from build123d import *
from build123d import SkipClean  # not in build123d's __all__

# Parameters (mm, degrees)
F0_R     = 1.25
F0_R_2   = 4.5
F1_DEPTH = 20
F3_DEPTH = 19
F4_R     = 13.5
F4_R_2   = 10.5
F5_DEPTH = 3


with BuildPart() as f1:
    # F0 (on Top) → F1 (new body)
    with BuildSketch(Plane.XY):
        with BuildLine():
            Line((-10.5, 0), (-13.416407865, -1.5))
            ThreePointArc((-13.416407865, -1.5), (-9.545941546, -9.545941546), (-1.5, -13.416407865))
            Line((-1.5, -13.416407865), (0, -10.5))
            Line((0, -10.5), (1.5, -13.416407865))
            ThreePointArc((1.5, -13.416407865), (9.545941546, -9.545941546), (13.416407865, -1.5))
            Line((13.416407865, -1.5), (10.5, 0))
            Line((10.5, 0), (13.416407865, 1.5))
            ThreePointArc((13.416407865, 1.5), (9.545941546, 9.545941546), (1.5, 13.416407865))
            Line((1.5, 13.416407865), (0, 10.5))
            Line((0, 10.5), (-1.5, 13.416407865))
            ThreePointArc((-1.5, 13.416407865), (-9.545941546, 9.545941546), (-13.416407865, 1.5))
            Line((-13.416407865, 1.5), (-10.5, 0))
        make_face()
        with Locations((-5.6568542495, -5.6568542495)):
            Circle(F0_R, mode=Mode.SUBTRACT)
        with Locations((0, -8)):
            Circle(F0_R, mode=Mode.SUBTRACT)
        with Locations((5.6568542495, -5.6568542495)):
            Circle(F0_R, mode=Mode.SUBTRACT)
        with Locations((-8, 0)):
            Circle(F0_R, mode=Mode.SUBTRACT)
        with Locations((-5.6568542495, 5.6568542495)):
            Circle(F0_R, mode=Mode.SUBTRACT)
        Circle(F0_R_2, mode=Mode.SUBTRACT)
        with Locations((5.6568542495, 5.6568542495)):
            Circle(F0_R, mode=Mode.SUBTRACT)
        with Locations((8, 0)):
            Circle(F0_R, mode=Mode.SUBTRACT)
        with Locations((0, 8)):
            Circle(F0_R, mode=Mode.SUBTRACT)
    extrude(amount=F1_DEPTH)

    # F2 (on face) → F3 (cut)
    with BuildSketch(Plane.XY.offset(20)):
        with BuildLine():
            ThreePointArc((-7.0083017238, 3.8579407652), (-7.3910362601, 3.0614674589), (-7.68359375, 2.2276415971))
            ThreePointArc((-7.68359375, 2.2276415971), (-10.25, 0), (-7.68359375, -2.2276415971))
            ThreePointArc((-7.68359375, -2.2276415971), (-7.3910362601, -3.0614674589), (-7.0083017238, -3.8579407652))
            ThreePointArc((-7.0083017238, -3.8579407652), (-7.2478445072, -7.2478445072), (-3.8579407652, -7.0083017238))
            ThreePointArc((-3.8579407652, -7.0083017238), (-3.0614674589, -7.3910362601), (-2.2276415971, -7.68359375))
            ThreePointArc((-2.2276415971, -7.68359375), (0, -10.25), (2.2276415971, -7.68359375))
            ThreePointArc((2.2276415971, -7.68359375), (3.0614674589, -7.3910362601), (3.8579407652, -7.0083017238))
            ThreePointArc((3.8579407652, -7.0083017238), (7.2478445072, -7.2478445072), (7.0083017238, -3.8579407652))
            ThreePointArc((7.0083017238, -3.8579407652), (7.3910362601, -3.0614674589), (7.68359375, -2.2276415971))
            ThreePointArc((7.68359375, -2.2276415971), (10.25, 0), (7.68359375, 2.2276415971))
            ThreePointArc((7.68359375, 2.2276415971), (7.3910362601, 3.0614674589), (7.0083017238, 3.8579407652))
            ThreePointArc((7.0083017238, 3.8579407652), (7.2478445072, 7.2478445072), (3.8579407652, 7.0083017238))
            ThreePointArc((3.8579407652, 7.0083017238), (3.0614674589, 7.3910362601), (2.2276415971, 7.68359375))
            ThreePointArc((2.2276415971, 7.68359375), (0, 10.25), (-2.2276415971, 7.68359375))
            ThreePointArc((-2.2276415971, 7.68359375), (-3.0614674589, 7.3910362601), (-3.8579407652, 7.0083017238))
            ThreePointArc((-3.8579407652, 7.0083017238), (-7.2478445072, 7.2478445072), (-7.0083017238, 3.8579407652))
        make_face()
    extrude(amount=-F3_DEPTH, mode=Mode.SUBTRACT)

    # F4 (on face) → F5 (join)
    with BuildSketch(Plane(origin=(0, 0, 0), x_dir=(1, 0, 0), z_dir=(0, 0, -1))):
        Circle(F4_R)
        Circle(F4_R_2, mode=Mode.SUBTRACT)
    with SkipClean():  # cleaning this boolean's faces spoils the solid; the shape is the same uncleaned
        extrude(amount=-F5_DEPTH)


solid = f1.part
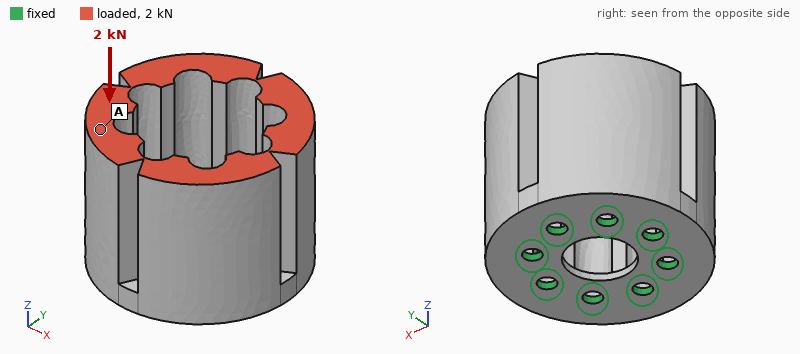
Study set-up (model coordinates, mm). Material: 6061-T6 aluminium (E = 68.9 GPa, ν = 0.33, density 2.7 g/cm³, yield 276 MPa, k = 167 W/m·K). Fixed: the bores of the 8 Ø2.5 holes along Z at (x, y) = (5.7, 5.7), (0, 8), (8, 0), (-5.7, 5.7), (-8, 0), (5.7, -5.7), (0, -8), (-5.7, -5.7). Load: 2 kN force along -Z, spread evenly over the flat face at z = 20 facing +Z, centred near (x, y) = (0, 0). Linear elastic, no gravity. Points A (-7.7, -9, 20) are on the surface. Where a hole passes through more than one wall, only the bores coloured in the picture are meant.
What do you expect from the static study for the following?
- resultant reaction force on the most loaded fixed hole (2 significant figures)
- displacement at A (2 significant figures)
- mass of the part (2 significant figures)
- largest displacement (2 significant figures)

260 N
6.1 µm
16 g
6.3 µm
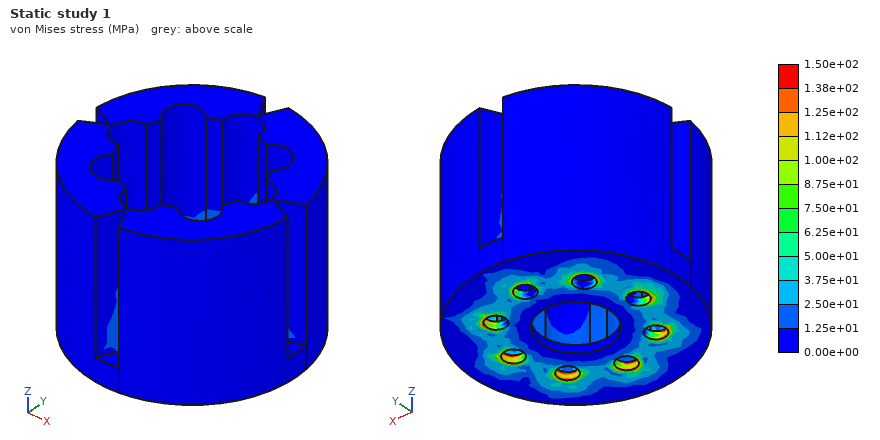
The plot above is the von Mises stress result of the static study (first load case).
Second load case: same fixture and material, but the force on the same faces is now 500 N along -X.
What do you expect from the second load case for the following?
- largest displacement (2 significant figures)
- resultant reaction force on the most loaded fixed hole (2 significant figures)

22 µm
270 N
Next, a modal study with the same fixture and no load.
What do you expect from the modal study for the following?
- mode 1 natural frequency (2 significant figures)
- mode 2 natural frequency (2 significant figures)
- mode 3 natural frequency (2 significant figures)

10 kHz
10 kHz
14 kHz
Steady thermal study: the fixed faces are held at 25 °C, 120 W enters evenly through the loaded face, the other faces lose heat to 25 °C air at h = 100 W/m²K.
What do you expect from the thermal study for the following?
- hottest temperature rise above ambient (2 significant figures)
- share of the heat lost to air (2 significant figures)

63 K
12 %
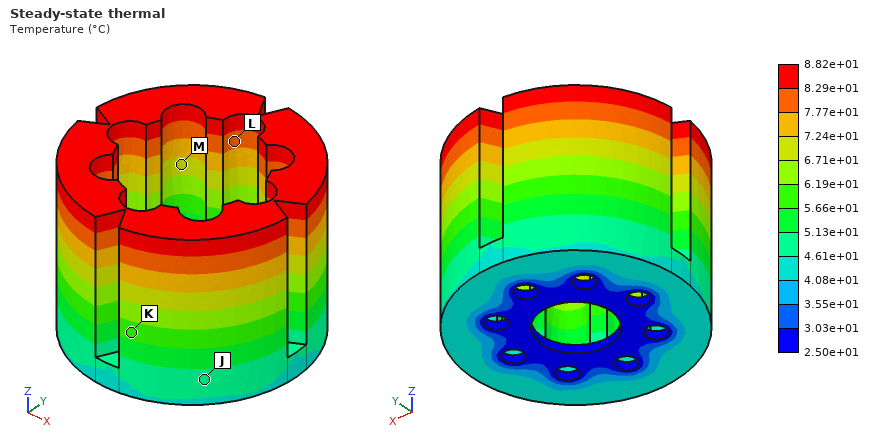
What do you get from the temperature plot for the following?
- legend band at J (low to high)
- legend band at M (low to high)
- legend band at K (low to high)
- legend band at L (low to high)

4.61e+01 to 5.13e+01 °C
6.71e+01 to 7.24e+01 °C
5.66e+01 to 6.19e+01 °C
7.77e+01 to 8.29e+01 °C
